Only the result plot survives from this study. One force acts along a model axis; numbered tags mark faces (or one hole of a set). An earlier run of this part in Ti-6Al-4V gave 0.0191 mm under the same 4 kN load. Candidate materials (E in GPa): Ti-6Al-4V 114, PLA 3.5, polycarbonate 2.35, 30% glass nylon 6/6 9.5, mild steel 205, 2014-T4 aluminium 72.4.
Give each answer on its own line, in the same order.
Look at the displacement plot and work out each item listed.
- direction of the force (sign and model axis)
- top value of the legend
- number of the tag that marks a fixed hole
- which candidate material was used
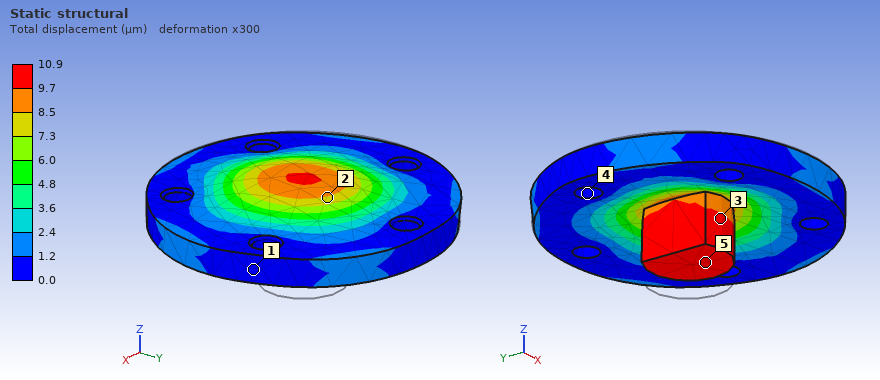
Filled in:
+Z
10.9 µm
4
mild steel
